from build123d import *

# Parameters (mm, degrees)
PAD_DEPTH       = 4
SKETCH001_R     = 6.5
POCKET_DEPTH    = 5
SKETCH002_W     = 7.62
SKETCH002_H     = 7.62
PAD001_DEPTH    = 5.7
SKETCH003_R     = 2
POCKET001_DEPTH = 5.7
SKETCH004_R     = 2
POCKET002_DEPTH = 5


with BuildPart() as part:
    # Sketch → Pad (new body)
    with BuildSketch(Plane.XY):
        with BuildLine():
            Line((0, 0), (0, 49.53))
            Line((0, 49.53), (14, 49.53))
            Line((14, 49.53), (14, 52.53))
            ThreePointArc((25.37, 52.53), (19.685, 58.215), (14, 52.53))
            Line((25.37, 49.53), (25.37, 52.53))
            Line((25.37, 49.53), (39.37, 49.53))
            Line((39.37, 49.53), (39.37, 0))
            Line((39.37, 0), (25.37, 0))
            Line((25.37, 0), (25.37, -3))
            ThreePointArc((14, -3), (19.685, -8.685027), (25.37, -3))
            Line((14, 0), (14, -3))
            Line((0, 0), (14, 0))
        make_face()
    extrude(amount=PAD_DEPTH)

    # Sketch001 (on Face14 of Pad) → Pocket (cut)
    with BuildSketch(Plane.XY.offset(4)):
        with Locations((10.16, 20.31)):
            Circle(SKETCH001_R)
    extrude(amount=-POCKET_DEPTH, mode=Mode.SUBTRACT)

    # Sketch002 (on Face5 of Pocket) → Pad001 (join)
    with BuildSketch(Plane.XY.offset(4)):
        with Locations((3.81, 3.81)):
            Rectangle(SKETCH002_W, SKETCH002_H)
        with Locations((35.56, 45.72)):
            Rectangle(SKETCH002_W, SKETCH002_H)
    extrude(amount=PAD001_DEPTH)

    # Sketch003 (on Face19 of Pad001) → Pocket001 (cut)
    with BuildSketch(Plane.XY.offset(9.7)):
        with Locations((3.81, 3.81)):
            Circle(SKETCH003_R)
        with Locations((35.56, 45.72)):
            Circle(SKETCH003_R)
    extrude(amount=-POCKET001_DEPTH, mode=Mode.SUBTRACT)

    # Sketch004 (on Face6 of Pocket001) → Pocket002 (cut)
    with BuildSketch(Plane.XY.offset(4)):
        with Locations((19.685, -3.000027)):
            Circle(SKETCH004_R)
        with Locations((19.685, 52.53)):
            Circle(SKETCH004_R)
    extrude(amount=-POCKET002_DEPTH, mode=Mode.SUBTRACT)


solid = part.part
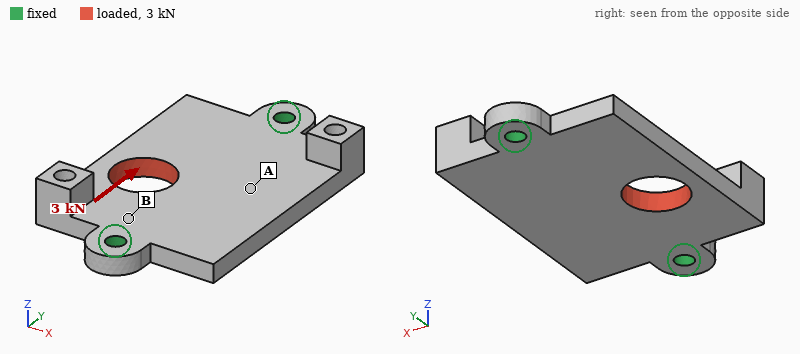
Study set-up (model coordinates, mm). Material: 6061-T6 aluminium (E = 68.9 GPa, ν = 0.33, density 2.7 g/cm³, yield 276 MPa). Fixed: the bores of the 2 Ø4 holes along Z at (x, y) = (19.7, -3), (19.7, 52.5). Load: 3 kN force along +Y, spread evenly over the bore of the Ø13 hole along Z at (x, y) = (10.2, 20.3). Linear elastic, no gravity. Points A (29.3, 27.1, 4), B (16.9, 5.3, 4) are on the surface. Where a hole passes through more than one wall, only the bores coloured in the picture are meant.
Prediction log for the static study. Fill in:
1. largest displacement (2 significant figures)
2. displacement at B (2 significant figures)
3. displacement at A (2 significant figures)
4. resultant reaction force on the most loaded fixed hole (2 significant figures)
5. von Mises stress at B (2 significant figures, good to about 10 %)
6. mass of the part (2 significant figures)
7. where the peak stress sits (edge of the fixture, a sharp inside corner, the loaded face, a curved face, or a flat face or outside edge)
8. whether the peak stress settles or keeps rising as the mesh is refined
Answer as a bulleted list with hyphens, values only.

- 18 µm
- 4.0 µm
- 4.2 µm
- 1.6 kN
- 30 MPa
- 23 g
- a sharp inside corner
- keeps rising
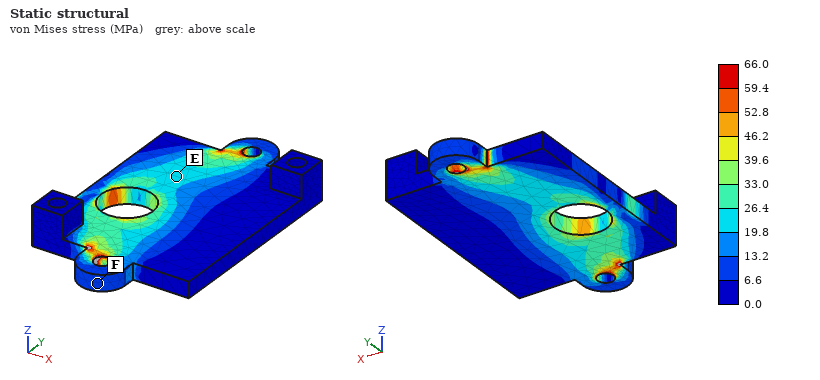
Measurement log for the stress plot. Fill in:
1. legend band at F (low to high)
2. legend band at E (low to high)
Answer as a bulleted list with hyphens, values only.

- 6.6 to 13.2 MPa
- 19.8 to 26.4 MPa
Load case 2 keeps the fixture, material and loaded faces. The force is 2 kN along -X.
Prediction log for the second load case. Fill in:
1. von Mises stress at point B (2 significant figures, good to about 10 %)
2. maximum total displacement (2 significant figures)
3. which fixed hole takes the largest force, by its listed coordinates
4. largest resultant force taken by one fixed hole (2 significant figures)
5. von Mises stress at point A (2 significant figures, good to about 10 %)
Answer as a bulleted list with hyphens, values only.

- 15 MPa
- 19 µm
- (19.7, -3)
- 1.2 kN
- 12 MPa
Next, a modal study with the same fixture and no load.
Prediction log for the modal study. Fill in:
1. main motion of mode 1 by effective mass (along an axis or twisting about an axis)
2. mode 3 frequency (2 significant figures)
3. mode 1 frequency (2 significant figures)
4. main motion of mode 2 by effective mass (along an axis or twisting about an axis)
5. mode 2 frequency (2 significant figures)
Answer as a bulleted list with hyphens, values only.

- twisting about Y
- 7600 Hz
- 3600 Hz
- along Z
- 4600 Hz
